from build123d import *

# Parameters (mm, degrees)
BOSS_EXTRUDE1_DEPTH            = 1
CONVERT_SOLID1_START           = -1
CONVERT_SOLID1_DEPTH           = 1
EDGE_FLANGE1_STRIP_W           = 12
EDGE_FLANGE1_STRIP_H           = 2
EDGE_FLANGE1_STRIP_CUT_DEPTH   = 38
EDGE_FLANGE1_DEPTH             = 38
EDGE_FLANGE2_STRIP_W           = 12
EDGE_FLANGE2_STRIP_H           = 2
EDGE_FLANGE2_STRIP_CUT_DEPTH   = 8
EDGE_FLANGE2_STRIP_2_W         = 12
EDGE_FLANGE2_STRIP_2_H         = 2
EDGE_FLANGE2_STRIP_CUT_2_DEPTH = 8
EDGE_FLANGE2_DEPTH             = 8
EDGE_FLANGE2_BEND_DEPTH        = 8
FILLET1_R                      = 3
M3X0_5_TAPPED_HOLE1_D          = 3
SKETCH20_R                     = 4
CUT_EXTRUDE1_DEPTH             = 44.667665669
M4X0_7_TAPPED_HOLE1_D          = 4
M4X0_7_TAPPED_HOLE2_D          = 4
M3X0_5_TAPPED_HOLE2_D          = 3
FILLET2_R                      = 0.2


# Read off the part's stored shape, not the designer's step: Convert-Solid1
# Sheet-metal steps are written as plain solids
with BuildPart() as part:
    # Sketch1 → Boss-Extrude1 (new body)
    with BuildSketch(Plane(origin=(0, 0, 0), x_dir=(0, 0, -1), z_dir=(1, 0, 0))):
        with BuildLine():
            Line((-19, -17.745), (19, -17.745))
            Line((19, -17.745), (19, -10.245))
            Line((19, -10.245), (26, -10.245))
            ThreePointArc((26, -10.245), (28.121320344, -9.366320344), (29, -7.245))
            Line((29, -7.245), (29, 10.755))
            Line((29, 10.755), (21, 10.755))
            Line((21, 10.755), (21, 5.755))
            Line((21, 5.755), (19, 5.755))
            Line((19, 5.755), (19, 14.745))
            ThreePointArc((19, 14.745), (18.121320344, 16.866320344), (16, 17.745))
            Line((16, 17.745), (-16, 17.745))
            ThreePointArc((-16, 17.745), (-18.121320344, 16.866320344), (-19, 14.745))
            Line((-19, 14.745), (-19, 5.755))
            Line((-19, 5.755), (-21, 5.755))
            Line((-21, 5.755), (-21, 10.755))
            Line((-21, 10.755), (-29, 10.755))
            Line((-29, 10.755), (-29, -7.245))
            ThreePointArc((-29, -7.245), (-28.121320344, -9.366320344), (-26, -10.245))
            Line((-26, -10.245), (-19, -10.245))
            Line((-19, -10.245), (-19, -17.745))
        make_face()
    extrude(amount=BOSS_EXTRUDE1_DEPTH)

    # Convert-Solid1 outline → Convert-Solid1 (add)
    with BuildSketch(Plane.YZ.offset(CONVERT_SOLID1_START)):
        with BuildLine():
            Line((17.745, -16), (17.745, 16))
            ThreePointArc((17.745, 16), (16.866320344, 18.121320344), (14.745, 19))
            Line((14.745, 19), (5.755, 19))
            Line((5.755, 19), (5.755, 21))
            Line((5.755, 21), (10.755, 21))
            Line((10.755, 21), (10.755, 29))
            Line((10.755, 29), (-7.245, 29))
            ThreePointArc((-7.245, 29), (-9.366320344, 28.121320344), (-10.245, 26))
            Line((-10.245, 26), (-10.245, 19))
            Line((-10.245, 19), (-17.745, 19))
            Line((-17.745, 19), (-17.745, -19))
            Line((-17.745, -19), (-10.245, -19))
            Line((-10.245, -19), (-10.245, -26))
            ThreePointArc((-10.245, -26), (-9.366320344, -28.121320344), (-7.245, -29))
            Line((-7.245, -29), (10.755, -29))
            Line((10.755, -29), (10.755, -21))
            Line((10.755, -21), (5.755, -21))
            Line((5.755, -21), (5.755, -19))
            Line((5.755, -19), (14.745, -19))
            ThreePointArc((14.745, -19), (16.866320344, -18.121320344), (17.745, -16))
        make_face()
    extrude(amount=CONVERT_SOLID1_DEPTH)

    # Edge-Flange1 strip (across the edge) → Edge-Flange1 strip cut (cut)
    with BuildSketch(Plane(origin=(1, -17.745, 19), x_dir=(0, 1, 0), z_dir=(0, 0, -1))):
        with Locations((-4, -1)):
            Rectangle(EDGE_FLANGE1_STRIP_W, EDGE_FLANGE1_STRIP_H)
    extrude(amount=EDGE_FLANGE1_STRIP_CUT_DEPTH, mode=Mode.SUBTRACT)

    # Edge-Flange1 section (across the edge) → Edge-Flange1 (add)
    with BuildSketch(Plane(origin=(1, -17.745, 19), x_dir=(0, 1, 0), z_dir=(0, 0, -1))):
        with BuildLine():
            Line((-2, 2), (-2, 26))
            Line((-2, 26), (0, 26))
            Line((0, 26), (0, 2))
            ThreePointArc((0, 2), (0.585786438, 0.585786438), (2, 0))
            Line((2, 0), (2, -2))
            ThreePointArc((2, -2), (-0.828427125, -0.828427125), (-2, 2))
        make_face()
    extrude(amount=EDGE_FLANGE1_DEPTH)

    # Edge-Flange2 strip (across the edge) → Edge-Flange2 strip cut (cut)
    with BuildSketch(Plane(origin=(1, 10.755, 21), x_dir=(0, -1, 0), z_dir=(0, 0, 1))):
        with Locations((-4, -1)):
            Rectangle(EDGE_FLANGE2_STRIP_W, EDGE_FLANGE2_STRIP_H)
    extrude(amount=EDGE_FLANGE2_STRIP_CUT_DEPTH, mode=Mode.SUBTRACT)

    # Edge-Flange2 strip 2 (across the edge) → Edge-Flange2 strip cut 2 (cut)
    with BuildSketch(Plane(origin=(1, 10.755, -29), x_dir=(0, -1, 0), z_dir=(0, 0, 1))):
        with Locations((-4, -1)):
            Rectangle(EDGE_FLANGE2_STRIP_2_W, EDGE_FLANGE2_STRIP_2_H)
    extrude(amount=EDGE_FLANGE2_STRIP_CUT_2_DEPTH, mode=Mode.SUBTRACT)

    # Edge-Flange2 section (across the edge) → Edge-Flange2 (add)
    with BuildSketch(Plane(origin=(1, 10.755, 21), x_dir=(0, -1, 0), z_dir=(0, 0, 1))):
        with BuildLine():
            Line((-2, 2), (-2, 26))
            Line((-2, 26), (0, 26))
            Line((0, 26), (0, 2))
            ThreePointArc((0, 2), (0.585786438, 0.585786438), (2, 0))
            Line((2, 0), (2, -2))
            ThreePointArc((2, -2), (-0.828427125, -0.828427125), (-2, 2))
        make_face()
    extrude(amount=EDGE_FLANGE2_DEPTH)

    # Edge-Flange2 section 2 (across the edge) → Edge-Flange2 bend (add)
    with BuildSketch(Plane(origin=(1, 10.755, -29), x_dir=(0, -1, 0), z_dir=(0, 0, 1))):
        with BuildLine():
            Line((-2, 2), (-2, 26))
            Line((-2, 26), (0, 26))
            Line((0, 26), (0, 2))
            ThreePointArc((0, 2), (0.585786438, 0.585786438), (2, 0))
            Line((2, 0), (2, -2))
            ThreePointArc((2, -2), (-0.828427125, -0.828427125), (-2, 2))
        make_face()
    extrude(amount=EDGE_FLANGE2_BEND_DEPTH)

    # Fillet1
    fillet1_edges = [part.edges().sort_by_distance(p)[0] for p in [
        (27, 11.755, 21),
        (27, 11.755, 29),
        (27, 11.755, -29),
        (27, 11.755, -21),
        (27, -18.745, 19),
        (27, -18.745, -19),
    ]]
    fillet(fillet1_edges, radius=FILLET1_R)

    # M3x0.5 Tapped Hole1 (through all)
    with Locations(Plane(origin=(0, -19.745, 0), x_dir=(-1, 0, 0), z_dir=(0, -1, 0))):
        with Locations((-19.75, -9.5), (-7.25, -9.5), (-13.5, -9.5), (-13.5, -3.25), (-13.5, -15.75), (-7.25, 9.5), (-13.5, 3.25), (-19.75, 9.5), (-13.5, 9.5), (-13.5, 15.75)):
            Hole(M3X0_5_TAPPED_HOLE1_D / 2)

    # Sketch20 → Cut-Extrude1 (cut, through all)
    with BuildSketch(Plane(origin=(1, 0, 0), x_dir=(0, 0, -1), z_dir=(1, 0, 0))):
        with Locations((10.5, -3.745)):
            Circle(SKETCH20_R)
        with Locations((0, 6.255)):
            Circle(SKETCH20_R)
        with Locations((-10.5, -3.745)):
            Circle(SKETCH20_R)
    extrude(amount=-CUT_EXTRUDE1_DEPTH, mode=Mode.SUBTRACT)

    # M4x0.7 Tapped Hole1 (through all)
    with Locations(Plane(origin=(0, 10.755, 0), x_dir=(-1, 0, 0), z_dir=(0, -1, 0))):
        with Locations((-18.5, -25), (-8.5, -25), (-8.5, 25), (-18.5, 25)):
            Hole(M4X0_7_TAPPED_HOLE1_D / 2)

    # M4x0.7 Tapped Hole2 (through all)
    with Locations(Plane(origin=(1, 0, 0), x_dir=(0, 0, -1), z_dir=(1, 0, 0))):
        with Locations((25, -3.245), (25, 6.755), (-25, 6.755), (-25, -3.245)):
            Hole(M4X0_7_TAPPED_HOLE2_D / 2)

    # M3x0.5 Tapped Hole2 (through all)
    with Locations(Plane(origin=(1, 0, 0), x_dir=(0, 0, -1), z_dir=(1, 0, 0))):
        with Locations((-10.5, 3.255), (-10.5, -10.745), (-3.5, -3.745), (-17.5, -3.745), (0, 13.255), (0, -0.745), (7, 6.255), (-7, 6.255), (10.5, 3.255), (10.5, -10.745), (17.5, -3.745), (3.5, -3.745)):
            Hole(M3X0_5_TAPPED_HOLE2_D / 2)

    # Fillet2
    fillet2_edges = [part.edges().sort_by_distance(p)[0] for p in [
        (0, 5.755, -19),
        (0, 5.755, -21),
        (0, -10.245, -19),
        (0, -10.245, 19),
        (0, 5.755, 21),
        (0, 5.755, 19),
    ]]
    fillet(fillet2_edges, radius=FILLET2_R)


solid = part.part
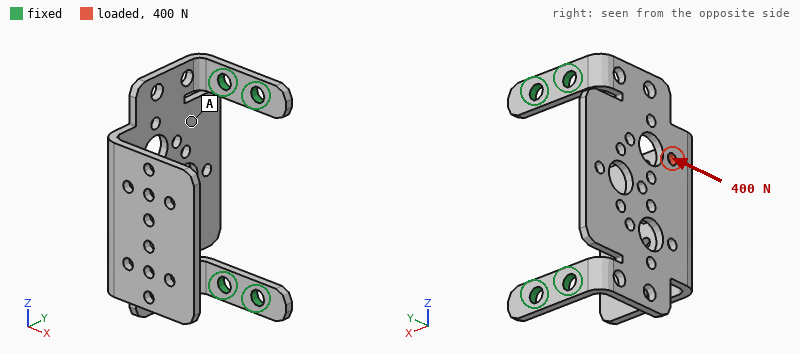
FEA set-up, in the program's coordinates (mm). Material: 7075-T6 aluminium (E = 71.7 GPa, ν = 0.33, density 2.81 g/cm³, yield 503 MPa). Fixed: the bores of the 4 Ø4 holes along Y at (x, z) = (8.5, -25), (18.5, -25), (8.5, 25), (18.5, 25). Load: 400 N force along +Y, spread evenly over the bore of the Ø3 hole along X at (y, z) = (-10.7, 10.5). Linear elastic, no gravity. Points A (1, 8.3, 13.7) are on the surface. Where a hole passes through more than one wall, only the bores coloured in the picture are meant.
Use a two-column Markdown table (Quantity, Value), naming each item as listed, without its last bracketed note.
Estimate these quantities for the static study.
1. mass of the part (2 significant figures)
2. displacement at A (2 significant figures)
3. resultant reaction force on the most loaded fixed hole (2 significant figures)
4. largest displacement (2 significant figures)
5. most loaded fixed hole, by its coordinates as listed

| Quantity | Value |
|---|---|
| mass of the part | 16 g |
| displacement at A | 0.087 mm |
| resultant reaction force on the most loaded fixed hole | 290 N |
| largest displacement | 0.51 mm |
| most loaded fixed hole, by its coordinates as listed | (8.5, 25) |
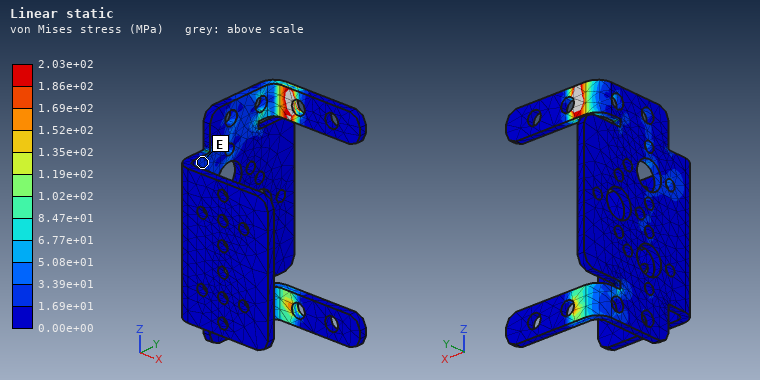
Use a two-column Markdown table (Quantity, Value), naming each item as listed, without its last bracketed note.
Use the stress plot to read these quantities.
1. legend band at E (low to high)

| Quantity | Value |
|---|---|
| legend band at E | 1.69e+01 to 3.39e+01 MPa |
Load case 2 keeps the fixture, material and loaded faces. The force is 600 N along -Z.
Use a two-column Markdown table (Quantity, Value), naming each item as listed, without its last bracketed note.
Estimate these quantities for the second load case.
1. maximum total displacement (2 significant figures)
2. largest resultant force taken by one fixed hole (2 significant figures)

| Quantity | Value |
|---|---|
| maximum total displacement | 0.29 mm |
| largest resultant force taken by one fixed hole | 420 N |
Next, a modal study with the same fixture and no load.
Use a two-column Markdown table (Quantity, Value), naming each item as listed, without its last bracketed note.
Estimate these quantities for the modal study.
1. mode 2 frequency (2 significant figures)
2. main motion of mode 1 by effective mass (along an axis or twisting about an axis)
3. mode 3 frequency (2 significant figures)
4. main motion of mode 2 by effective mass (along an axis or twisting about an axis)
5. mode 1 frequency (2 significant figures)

| Quantity | Value |
|---|---|
| mode 2 frequency | 1100 Hz |
| main motion of mode 1 by effective mass | along X |
| mode 3 frequency | 1400 Hz |
| main motion of mode 2 by effective mass | along Z |
| mode 1 frequency | 360 Hz |
